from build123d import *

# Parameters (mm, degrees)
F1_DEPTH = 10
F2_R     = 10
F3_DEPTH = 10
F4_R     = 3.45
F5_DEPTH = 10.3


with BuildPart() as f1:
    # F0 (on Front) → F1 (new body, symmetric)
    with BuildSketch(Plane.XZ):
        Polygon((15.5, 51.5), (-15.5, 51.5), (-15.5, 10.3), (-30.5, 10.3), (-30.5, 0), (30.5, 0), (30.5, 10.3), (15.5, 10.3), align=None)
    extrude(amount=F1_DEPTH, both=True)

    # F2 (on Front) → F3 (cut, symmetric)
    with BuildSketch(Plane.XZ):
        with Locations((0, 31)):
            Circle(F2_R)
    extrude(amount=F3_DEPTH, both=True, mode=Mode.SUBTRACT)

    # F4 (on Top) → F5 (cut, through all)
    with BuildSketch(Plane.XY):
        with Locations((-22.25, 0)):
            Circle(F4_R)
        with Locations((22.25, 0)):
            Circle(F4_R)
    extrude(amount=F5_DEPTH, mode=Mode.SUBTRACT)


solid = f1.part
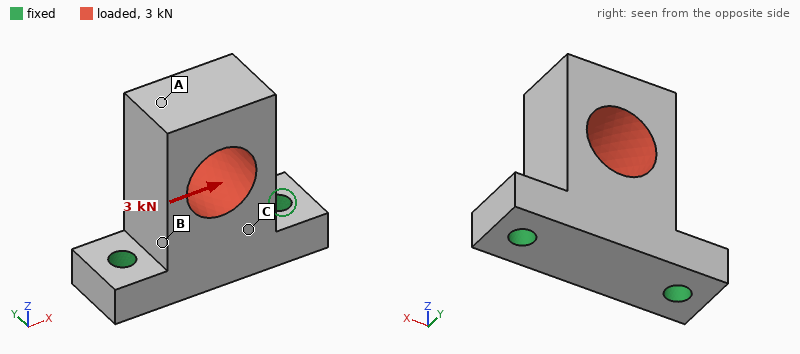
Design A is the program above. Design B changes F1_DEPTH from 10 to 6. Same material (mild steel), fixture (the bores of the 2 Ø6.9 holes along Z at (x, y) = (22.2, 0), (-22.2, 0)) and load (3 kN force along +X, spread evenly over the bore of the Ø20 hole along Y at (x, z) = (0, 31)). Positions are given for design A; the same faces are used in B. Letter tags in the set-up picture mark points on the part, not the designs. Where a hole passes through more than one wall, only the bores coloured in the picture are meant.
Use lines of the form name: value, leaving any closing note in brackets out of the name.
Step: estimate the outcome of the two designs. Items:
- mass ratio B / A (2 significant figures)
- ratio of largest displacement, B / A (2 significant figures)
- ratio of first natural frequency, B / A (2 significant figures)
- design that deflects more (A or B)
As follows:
mass ratio B / A: 0.59
ratio of largest displacement, B / A: 1.6
ratio of first natural frequency, B / A: 0.79
design that deflects more: B
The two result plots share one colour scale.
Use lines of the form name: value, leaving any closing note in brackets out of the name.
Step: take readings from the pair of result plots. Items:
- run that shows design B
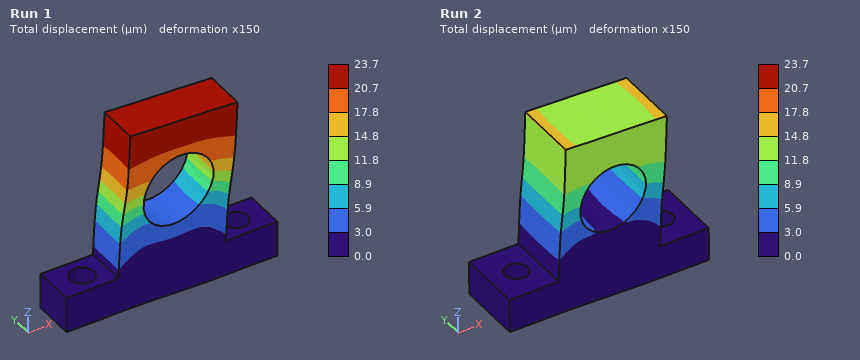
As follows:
run that shows design B: Run 1
